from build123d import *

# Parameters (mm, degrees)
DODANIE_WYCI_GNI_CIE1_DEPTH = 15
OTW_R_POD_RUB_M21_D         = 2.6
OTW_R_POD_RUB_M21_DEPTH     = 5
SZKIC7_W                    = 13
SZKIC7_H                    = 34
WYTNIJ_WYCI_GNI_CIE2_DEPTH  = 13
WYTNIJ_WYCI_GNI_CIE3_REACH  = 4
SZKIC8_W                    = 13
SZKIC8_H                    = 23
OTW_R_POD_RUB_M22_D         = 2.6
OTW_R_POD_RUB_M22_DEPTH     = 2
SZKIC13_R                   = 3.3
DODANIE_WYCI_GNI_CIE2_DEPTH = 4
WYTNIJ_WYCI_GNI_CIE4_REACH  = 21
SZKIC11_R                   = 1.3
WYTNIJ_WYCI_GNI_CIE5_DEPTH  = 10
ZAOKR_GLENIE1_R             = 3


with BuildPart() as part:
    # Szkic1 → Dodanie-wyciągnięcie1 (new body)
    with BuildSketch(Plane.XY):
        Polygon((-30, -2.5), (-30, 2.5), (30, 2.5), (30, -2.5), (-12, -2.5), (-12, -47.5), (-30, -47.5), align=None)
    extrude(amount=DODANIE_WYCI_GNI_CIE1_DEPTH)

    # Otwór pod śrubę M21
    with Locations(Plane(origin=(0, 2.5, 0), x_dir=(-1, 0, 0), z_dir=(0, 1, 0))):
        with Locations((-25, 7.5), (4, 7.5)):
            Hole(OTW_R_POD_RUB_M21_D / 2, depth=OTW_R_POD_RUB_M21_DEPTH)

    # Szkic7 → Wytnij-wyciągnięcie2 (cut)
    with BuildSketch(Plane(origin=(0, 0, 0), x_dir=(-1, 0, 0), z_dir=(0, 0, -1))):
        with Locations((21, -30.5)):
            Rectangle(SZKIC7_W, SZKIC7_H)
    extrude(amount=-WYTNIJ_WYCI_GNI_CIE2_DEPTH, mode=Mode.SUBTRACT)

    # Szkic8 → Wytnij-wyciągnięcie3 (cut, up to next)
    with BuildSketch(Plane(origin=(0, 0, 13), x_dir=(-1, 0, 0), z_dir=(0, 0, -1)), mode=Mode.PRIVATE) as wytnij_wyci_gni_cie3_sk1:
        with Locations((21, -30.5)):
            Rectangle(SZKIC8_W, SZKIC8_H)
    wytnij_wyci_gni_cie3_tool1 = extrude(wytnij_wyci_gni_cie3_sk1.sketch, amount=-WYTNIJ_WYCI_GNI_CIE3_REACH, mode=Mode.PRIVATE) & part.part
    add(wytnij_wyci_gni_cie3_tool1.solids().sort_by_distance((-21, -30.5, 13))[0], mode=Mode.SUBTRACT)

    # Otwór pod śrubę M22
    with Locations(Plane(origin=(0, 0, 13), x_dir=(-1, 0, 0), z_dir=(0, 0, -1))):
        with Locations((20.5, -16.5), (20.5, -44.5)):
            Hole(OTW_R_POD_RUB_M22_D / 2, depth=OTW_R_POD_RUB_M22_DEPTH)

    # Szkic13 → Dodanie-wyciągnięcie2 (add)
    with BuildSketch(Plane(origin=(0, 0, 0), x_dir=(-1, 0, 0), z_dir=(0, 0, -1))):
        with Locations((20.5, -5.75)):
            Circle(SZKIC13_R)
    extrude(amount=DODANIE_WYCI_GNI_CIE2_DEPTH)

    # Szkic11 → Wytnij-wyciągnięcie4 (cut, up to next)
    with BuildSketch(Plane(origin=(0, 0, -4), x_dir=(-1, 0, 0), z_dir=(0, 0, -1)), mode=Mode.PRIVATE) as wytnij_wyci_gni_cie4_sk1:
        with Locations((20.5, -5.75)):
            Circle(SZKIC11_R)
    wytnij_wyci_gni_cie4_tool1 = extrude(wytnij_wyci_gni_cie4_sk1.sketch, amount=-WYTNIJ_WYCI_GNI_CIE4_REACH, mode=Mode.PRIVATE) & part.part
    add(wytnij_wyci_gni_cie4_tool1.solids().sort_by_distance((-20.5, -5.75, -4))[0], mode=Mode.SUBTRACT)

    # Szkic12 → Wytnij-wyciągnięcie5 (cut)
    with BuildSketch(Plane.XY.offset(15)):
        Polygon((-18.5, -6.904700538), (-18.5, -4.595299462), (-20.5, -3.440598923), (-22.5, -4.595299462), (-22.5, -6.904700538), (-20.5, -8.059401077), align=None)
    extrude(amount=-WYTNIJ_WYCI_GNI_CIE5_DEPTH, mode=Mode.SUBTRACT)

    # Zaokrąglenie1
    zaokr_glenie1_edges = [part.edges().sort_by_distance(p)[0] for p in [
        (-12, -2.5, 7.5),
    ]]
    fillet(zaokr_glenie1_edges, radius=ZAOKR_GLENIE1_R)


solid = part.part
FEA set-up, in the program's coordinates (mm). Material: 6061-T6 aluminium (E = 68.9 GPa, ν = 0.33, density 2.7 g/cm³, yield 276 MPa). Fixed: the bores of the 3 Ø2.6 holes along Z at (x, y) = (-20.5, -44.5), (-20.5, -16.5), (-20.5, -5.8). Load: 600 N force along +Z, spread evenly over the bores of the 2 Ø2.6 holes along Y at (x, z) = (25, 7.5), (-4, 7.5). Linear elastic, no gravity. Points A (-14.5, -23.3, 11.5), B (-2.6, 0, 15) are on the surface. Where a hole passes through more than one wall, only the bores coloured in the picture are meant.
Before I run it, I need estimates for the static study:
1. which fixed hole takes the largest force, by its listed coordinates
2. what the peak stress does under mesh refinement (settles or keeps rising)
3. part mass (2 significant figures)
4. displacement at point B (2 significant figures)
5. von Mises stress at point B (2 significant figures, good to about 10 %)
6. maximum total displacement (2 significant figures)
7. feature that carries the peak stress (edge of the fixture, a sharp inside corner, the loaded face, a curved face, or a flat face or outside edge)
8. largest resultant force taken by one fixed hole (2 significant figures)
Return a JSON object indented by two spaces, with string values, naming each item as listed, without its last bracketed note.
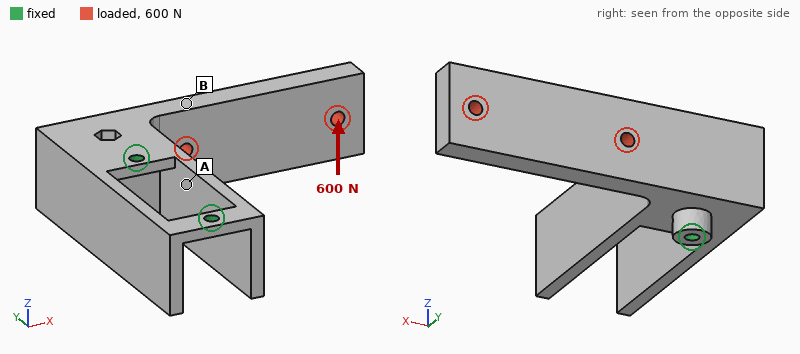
{
  "which fixed hole takes the largest force, by its listed coordinates": "(-20.5, -5.8)",
  "what the peak stress does under mesh refinement": "keeps rising",
  "part mass": "28 g",
  "displacement at point B": "0.071 mm",
  "von Mises stress at point B": "42 MPa",
  "maximum total displacement": "0.22 mm",
  "feature that carries the peak stress": "edge of the fixture",
  "largest resultant force taken by one fixed hole": "910 N"
}
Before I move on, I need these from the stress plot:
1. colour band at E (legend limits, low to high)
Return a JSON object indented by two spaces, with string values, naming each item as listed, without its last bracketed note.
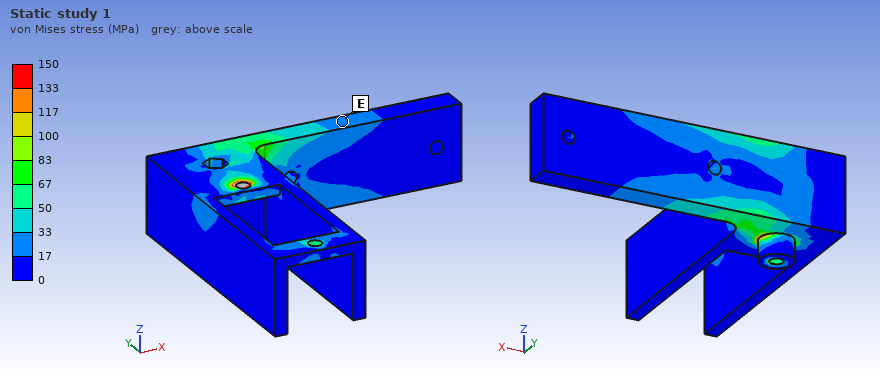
{
  "colour band at E": "17 to 33 MPa"
}
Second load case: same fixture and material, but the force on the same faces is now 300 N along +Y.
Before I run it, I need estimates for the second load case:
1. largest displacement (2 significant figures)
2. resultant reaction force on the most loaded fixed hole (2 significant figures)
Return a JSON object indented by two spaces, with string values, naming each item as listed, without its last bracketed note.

{
  "largest displacement": "0.41 mm",
  "resultant reaction force on the most loaded fixed hole": "360 N"
}
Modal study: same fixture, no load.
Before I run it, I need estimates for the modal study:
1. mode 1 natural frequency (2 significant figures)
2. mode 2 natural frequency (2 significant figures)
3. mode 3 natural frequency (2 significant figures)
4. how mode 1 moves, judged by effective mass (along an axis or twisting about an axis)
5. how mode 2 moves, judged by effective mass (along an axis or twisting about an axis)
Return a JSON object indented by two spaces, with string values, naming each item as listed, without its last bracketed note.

{
  "mode 1 natural frequency": "2000 Hz",
  "mode 2 natural frequency": "3800 Hz",
  "mode 3 natural frequency": "6000 Hz",
  "how mode 1 moves, judged by effective mass": "along Y",
  "how mode 2 moves, judged by effective mass": "along Z"
}
